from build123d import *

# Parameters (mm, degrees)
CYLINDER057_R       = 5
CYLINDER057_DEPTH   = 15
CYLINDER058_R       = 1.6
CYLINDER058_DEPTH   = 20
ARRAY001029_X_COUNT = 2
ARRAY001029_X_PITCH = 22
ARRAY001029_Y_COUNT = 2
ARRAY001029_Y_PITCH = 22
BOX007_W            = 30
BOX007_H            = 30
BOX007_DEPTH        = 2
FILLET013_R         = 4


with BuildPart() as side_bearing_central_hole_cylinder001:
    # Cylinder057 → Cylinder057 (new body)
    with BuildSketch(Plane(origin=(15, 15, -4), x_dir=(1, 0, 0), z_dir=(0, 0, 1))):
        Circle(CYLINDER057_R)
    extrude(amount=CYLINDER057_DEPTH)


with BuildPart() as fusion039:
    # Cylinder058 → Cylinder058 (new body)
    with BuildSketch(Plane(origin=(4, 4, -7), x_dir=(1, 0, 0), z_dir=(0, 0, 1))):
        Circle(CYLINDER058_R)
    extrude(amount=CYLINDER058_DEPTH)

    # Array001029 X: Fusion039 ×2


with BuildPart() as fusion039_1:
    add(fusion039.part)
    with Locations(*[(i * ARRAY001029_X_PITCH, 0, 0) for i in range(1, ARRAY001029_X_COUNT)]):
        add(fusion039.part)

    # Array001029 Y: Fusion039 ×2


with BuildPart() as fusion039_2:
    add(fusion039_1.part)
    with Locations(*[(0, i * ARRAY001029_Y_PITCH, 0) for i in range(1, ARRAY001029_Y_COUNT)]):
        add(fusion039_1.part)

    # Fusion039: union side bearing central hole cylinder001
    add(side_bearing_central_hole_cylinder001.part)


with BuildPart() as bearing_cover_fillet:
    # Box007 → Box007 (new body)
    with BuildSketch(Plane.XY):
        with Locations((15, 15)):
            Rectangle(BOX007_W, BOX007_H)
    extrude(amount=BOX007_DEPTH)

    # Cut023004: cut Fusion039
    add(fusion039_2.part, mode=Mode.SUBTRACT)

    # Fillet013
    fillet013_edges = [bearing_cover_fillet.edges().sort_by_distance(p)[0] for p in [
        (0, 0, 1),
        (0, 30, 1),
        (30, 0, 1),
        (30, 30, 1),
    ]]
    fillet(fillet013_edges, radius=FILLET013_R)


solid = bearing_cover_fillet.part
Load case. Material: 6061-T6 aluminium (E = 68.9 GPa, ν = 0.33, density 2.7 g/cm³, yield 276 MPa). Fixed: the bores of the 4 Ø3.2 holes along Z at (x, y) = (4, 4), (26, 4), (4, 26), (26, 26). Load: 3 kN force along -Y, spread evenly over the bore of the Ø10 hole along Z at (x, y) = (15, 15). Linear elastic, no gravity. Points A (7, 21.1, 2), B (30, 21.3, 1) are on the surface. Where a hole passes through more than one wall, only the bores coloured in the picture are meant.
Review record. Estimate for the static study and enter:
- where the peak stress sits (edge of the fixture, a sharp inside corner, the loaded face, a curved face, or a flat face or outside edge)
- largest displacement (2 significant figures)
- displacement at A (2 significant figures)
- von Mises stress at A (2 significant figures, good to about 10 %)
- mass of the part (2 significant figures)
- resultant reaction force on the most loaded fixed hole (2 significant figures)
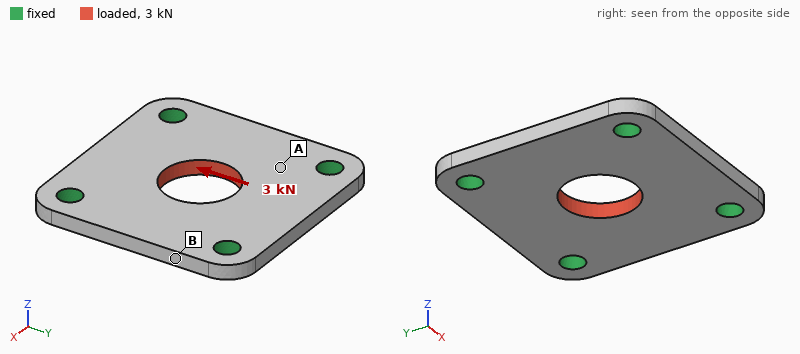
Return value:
edge of the fixture
12 µm
4.1 µm
50 MPa
4.2 g
810 N
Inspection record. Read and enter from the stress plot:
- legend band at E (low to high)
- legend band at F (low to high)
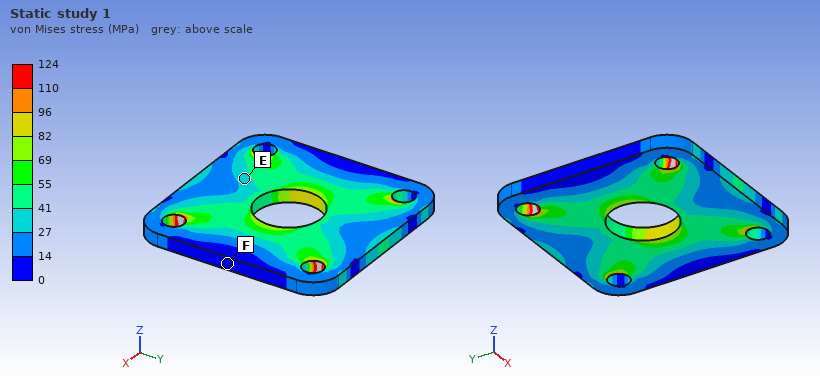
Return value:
27 to 41 MPa
0 to 14 MPa
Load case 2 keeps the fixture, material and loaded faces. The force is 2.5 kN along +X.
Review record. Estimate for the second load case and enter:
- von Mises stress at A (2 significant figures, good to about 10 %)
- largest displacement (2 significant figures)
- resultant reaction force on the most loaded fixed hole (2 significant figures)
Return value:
43 MPa
9.9 µm
680 N
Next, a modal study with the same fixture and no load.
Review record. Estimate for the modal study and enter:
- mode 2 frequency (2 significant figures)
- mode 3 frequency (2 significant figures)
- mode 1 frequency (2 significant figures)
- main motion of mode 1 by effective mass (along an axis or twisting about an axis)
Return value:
25 kHz
25 kHz
19 kHz
along Z
